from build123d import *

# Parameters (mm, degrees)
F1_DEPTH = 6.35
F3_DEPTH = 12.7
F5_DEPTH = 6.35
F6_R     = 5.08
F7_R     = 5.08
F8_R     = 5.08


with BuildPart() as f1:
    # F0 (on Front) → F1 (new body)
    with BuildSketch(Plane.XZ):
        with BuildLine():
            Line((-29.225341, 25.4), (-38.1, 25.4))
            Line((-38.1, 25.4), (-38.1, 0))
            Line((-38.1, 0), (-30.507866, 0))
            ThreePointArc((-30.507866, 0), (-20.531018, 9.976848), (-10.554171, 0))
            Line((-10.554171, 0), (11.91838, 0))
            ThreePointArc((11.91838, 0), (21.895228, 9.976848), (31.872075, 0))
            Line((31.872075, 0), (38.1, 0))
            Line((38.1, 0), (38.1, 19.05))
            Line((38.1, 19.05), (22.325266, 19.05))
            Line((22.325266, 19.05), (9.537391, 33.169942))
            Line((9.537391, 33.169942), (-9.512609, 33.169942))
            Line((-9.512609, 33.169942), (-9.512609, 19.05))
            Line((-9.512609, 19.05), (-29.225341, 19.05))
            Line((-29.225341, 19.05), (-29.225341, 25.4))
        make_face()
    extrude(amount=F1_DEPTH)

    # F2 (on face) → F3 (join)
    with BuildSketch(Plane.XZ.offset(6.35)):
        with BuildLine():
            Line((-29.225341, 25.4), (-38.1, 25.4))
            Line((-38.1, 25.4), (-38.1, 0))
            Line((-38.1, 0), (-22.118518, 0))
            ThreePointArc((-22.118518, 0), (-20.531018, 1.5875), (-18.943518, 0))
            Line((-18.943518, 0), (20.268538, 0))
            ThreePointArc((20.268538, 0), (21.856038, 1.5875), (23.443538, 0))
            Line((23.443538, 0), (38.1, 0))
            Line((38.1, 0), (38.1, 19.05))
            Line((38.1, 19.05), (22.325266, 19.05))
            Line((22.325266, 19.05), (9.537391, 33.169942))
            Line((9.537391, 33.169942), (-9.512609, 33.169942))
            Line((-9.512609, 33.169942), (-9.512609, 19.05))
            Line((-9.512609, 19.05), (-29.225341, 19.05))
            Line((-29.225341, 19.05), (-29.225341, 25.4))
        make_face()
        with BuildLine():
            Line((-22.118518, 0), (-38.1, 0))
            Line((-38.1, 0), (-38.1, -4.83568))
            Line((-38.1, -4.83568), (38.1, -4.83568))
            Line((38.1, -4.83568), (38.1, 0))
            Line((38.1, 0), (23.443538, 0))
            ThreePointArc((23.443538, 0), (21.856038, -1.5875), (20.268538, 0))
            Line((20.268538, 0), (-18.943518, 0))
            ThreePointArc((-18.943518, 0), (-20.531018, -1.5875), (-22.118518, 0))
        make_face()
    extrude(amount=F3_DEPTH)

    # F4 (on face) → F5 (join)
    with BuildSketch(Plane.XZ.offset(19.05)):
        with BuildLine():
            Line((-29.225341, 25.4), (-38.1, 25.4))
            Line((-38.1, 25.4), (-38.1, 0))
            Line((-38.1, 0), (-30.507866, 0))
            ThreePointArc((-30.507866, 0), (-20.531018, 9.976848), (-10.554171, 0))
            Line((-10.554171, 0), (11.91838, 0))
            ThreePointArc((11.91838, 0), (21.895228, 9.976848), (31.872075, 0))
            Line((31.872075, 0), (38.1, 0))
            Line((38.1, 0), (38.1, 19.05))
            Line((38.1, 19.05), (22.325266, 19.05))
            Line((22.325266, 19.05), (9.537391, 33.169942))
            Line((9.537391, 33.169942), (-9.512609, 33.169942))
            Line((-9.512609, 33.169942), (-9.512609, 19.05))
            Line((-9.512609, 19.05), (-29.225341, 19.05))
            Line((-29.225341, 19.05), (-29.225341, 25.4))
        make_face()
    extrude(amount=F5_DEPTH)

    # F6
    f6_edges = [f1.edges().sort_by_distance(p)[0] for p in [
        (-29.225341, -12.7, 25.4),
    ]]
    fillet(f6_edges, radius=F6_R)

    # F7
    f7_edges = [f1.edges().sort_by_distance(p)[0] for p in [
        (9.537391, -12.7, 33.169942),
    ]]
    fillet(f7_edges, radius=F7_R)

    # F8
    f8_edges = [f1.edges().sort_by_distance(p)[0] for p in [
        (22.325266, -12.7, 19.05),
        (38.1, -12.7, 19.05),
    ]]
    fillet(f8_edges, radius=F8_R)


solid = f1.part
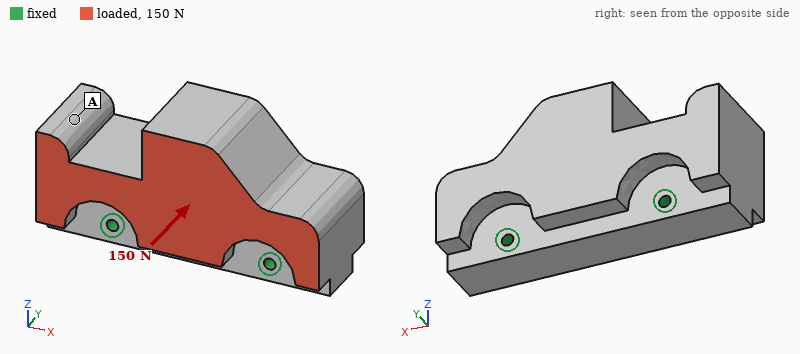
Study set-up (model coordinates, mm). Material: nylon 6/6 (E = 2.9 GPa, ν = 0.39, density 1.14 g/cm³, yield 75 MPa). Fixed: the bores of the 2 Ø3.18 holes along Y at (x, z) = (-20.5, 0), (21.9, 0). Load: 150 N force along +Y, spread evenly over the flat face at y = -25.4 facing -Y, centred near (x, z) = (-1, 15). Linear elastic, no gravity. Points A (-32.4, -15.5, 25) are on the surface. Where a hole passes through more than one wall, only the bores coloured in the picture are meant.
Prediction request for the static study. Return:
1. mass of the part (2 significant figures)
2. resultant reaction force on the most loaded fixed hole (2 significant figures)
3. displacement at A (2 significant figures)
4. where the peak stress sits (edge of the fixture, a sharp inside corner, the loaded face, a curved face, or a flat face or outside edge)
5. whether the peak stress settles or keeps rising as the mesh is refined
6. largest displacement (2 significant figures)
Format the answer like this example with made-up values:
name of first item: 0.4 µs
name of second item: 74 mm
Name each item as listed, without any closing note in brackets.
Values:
mass of the part: 54 g
resultant reaction force on the most loaded fixed hole: 78 N
displacement at A: 29 µm
where the peak stress sits: edge of the fixture
whether the peak stress settles or keeps rising as the mesh is refined: keeps rising
largest displacement: 45 µm
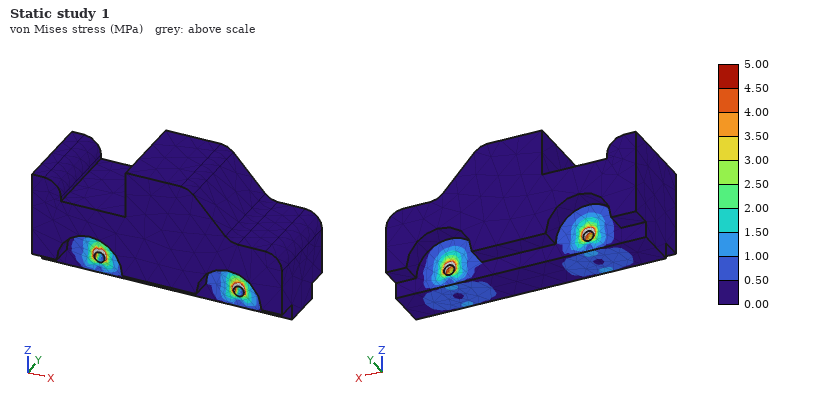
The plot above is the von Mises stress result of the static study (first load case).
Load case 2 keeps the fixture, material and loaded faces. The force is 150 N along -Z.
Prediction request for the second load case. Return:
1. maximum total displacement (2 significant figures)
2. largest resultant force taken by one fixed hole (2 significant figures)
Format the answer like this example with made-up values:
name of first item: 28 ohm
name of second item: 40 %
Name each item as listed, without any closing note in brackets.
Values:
maximum total displacement: 43 µm
largest resultant force taken by one fixed hole: 80 N
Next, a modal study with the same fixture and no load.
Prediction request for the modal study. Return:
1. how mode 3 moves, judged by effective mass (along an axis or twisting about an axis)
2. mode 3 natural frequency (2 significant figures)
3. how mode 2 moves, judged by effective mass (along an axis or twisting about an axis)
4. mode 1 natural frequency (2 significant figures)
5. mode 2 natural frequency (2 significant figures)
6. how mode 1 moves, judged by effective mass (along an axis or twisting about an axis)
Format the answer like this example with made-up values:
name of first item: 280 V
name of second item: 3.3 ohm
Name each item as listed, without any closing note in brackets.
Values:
how mode 3 moves, judged by effective mass: along X
mode 3 natural frequency: 4000 Hz
how mode 2 moves, judged by effective mass: twisting about Z
mode 1 natural frequency: 1700 Hz
mode 2 natural frequency: 3500 Hz
how mode 1 moves, judged by effective mass: along Y
